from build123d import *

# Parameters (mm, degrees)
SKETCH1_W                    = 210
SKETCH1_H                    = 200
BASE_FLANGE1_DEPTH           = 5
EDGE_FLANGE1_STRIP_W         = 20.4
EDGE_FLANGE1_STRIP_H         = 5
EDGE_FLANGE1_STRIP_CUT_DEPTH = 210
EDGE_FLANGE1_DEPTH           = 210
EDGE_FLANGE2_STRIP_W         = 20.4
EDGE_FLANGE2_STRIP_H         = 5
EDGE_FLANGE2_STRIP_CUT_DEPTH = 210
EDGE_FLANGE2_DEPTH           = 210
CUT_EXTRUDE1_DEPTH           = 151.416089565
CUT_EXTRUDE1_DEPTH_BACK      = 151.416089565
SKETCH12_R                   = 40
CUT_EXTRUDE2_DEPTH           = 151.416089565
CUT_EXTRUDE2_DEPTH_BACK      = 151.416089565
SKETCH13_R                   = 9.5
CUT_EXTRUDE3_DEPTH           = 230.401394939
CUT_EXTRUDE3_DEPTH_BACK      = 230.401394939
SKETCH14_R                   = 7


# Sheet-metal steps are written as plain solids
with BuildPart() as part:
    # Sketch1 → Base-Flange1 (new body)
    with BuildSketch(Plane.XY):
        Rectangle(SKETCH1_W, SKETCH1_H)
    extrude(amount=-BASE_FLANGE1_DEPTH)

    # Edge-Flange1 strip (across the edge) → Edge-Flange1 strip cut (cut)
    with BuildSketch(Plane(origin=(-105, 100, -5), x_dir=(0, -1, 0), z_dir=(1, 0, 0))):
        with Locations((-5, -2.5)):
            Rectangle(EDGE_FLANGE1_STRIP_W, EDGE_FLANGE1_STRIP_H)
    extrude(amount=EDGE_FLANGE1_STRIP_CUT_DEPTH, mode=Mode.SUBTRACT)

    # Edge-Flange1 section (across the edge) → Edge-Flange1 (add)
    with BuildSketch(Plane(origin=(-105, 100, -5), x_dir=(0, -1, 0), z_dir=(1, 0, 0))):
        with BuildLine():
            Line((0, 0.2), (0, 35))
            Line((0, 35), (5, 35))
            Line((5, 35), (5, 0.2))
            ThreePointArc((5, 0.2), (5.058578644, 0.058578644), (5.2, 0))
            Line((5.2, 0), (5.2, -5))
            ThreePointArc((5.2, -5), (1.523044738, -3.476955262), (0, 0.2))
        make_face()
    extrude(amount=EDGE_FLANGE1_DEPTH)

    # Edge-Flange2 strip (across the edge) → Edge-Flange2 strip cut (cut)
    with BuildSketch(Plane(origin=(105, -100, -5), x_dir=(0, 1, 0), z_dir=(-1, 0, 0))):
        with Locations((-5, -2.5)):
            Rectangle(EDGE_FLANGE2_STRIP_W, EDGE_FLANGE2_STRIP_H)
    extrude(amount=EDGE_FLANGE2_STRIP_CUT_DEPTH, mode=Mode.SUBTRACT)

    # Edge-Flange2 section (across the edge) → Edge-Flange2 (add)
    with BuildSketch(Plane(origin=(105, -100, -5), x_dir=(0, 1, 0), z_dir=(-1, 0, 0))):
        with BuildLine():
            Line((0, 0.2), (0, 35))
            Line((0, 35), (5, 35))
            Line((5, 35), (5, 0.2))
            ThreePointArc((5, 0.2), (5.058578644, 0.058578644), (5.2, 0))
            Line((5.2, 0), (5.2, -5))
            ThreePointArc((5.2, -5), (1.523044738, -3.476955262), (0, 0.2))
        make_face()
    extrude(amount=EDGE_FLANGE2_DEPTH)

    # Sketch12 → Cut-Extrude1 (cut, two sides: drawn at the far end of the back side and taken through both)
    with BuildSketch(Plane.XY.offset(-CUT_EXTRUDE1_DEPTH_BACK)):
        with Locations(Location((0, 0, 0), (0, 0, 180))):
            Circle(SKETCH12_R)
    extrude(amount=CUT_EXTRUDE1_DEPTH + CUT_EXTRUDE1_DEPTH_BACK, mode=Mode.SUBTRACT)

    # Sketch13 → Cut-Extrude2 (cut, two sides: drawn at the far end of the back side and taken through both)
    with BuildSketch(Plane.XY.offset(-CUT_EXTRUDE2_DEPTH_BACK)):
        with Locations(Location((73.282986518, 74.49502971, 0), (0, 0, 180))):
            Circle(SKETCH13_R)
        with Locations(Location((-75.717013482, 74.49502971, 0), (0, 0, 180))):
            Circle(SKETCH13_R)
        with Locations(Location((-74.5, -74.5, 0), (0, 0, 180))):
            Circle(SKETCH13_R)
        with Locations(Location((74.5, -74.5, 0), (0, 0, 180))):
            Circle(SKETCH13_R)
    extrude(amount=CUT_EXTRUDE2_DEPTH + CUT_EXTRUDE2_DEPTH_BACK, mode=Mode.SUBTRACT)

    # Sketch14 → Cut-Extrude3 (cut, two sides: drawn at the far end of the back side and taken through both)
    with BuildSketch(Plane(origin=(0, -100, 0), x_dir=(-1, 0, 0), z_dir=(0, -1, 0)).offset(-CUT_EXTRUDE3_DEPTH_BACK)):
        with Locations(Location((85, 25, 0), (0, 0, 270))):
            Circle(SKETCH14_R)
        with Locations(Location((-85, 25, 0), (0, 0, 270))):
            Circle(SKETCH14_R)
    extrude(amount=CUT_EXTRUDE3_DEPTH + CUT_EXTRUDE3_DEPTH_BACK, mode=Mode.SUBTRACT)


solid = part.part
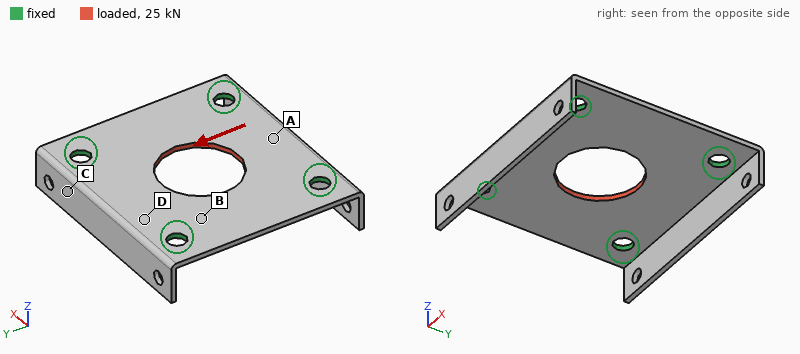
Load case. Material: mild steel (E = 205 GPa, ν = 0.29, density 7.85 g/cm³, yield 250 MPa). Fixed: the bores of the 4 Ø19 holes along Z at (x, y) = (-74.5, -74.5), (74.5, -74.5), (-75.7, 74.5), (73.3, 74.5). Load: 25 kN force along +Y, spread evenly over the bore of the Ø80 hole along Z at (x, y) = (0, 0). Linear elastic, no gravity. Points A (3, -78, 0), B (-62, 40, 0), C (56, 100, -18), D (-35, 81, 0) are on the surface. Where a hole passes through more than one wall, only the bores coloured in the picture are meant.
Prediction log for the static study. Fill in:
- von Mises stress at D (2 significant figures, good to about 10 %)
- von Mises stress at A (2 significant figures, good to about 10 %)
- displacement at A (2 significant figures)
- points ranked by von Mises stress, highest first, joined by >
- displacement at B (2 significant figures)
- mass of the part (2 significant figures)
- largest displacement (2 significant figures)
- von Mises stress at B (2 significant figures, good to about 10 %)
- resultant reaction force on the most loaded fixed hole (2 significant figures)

15 MPa
9.1 MPa
11 µm
B > D > A > C
4.0 µm
1.9 kg
13 µm
21 MPa
6.7 kN
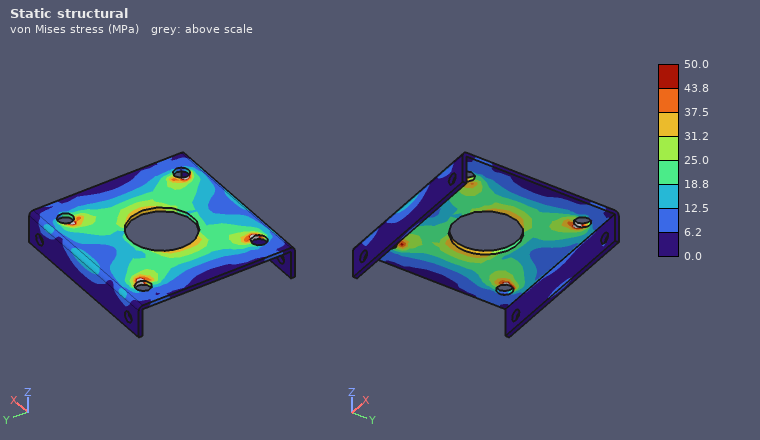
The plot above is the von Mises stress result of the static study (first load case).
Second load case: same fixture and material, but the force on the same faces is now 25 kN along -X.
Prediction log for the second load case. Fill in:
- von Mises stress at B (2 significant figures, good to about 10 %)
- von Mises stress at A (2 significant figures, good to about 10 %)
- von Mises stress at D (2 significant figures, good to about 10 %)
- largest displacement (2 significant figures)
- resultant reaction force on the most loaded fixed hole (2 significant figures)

22 MPa
11 MPa
12 MPa
13 µm
6.7 kN
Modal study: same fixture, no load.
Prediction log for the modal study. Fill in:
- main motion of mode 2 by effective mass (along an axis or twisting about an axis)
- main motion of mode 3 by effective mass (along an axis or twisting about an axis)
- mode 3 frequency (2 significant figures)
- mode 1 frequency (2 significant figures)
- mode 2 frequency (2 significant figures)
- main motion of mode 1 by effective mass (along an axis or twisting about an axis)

twisting about Y
along Y
1500 Hz
1200 Hz
1400 Hz
along Z
